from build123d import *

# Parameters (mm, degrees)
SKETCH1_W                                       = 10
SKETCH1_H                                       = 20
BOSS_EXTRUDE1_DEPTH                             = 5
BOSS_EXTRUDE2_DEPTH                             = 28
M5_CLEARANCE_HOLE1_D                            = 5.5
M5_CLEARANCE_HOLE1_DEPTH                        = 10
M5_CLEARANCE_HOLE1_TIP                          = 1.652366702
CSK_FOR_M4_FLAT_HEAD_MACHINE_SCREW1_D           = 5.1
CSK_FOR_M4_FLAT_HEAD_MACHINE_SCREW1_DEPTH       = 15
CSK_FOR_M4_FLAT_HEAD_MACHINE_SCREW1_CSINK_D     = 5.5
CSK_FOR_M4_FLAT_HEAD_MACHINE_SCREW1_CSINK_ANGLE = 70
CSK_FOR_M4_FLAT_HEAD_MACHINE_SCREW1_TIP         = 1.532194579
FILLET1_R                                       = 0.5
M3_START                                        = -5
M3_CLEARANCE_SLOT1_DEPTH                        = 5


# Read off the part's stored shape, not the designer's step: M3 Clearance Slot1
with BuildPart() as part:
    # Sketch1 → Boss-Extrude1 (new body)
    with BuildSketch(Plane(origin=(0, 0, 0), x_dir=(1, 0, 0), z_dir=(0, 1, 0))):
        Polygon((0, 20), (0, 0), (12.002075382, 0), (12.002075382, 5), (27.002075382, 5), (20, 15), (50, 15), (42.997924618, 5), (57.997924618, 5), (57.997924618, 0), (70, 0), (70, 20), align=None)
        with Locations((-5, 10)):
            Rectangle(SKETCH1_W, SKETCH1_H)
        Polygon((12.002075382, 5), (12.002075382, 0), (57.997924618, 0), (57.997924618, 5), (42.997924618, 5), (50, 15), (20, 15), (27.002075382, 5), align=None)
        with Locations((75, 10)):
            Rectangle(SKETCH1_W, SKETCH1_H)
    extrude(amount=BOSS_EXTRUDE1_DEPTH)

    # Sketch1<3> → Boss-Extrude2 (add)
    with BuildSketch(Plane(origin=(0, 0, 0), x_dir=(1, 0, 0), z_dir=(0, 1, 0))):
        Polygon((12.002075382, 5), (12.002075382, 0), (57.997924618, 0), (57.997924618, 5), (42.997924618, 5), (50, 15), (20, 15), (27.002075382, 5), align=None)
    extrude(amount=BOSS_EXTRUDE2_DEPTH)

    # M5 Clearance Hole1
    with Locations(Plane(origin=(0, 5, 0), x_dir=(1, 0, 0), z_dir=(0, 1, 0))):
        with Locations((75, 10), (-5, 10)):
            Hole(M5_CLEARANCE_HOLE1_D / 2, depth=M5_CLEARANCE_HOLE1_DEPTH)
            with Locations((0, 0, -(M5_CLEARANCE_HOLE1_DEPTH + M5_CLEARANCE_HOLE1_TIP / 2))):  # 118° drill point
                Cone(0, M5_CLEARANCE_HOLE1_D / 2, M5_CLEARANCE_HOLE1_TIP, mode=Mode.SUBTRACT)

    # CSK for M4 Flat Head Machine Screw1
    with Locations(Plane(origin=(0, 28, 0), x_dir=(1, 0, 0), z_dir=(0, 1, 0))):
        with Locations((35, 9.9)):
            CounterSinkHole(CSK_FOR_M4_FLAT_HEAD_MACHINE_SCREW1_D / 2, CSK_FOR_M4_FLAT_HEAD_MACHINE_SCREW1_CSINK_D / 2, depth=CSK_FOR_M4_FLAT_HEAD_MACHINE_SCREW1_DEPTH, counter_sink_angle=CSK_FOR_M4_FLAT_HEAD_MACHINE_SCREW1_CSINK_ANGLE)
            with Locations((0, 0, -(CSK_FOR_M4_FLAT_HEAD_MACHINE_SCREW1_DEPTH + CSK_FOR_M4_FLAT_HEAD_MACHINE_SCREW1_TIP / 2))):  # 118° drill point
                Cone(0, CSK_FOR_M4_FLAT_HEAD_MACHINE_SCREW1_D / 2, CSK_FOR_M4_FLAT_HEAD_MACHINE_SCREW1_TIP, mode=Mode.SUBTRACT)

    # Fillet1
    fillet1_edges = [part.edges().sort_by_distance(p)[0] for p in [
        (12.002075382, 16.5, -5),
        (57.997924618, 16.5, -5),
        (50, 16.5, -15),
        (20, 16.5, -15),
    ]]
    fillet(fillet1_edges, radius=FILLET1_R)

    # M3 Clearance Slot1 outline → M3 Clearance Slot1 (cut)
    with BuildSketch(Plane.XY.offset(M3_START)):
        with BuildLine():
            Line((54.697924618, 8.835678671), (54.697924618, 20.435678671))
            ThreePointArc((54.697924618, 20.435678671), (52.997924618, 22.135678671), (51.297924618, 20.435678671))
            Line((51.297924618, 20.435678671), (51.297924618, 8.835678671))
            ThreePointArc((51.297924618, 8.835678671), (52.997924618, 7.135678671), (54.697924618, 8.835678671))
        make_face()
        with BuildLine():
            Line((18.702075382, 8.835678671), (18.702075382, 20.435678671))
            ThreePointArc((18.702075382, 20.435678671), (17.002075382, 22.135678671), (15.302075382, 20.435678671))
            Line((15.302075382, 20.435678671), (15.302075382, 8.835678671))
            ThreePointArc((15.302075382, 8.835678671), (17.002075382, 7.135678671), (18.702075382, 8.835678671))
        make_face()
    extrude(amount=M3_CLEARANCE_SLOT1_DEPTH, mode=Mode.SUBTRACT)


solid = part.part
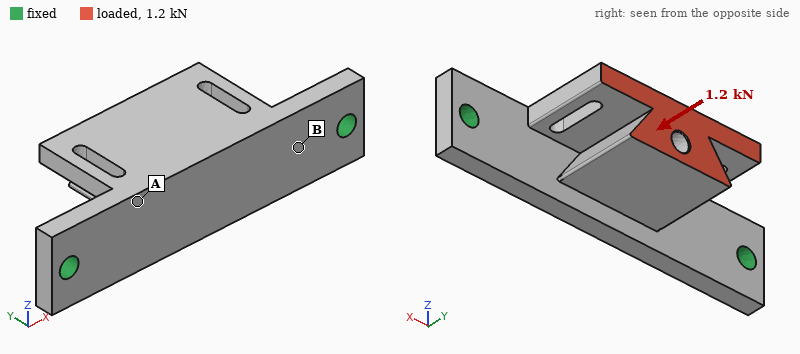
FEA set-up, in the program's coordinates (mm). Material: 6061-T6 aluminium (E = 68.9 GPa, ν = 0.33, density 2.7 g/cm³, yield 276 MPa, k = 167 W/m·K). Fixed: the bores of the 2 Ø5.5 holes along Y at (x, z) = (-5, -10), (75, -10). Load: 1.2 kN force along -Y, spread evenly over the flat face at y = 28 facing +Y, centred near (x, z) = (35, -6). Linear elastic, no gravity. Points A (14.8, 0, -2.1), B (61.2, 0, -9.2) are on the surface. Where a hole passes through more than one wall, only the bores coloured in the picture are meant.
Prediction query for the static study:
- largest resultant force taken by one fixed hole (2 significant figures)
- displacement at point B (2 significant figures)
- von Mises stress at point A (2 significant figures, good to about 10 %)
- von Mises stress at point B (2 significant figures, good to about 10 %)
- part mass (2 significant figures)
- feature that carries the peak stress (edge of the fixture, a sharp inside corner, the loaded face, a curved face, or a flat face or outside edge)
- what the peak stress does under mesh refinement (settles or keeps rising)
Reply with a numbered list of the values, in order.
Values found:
1. 670 N
2. 31 µm
3. 44 MPa
4. 17 MPa
5. 50 g
6. a sharp inside corner
7. keeps rising
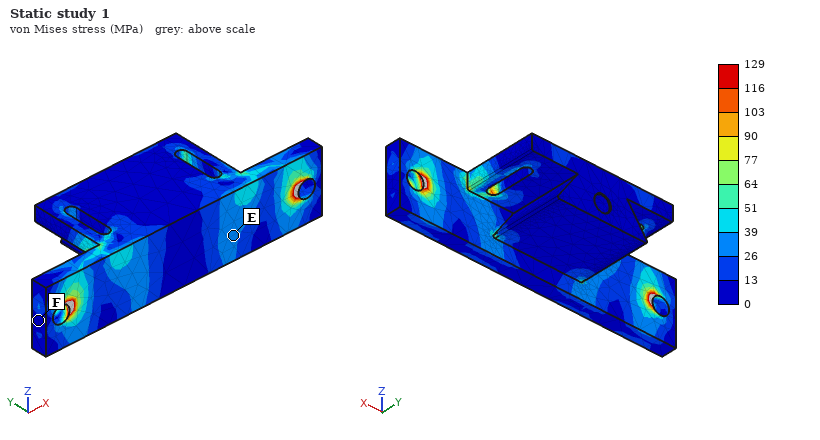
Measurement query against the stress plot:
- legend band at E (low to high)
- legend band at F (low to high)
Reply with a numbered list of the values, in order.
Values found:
1. 26 to 39 MPa
2. 0 to 13 MPa
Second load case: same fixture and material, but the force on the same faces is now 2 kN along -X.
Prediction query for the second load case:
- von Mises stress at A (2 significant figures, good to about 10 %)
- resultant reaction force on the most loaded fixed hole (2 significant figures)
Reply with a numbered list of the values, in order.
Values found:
1. 76 MPa
2. 1.3 kN
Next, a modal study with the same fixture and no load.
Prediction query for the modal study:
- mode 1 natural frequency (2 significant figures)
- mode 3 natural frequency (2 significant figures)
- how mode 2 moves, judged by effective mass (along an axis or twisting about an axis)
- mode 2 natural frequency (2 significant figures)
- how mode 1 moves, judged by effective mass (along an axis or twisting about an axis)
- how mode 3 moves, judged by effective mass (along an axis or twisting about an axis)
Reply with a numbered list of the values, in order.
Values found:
1. 2300 Hz
2. 6100 Hz
3. along Y
4. 3600 Hz
5. along Z
6. along X
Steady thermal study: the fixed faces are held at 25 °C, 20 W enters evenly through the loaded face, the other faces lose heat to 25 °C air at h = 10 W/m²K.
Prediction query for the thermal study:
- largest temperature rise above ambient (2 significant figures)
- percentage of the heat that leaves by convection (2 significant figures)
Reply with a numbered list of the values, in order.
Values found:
1. 22 K
2. 5.0 %
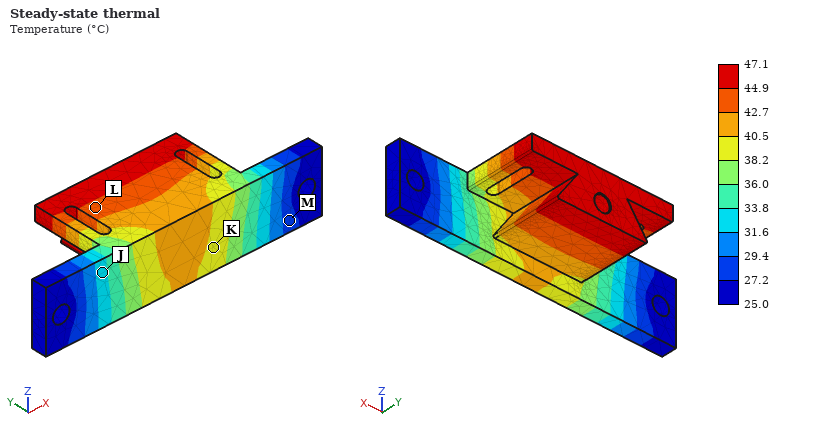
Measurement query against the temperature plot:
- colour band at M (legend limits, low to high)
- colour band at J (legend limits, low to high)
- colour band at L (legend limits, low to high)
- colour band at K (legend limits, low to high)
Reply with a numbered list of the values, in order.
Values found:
1. 27.2 to 29.4 °C
2. 31.6 to 33.8 °C
3. 42.7 to 44.9 °C
4. 38.2 to 40.5 °C
